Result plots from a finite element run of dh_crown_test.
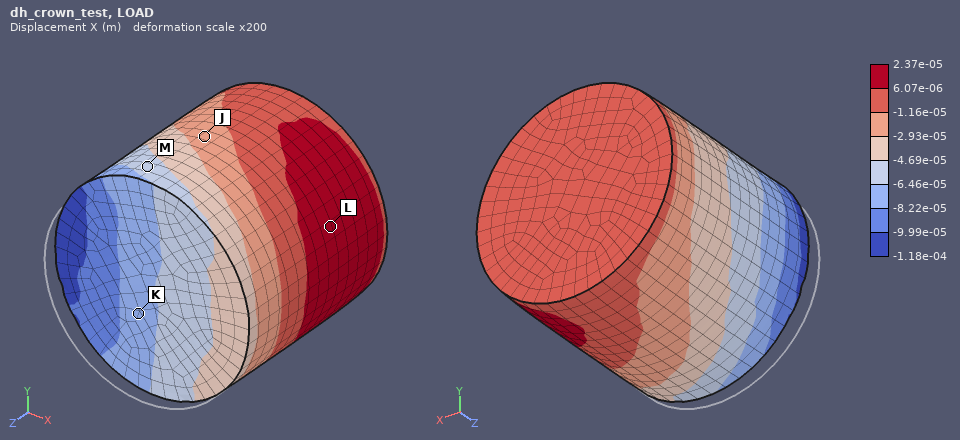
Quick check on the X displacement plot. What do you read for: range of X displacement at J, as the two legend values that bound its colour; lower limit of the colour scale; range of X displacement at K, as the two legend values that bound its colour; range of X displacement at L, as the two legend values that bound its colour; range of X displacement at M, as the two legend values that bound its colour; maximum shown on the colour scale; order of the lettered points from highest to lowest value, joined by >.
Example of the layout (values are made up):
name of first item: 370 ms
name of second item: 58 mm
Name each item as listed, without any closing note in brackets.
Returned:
range of X displacement at J, as the two legend values that bound its colour: -2.93e-05 to -1.16e-05 m
lower limit of the colour scale: -1.18e-04 m
range of X displacement at K, as the two legend values that bound its colour: -8.22e-05 to -6.46e-05 m
range of X displacement at L, as the two legend values that bound its colour: 6.07e-06 to 2.37e-05 m
range of X displacement at M, as the two legend values that bound its colour: -6.46e-05 to -4.69e-05 m
maximum shown on the colour scale: 2.37e-05 m
order of the lettered points from highest to lowest value, joined by >: L > J > M > K
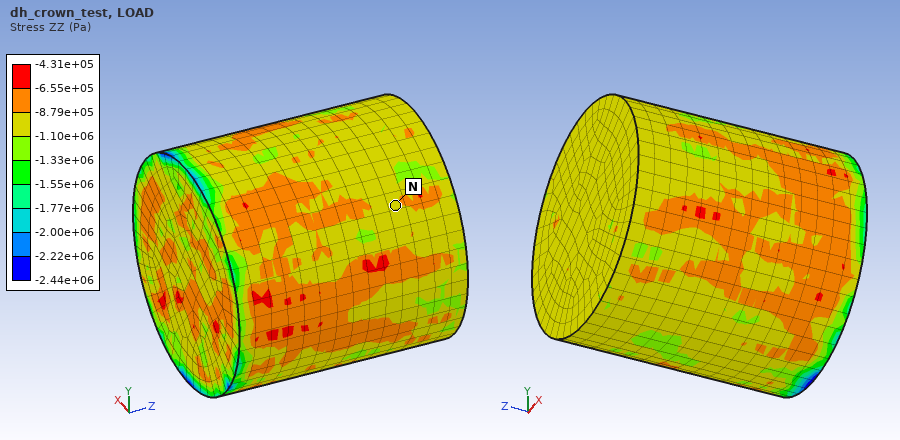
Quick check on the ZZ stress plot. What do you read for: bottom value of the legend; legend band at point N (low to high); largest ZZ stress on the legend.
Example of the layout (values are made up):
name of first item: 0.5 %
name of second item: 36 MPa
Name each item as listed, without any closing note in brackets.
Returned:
bottom value of the legend: -2.44e+06 Pa
legend band at point N: -1.10e+06 to -8.79e+05 Pa
largest ZZ stress on the legend: -4.31e+05 Pa
